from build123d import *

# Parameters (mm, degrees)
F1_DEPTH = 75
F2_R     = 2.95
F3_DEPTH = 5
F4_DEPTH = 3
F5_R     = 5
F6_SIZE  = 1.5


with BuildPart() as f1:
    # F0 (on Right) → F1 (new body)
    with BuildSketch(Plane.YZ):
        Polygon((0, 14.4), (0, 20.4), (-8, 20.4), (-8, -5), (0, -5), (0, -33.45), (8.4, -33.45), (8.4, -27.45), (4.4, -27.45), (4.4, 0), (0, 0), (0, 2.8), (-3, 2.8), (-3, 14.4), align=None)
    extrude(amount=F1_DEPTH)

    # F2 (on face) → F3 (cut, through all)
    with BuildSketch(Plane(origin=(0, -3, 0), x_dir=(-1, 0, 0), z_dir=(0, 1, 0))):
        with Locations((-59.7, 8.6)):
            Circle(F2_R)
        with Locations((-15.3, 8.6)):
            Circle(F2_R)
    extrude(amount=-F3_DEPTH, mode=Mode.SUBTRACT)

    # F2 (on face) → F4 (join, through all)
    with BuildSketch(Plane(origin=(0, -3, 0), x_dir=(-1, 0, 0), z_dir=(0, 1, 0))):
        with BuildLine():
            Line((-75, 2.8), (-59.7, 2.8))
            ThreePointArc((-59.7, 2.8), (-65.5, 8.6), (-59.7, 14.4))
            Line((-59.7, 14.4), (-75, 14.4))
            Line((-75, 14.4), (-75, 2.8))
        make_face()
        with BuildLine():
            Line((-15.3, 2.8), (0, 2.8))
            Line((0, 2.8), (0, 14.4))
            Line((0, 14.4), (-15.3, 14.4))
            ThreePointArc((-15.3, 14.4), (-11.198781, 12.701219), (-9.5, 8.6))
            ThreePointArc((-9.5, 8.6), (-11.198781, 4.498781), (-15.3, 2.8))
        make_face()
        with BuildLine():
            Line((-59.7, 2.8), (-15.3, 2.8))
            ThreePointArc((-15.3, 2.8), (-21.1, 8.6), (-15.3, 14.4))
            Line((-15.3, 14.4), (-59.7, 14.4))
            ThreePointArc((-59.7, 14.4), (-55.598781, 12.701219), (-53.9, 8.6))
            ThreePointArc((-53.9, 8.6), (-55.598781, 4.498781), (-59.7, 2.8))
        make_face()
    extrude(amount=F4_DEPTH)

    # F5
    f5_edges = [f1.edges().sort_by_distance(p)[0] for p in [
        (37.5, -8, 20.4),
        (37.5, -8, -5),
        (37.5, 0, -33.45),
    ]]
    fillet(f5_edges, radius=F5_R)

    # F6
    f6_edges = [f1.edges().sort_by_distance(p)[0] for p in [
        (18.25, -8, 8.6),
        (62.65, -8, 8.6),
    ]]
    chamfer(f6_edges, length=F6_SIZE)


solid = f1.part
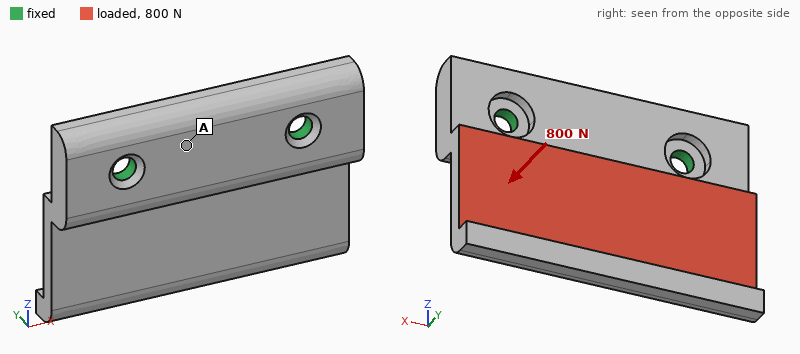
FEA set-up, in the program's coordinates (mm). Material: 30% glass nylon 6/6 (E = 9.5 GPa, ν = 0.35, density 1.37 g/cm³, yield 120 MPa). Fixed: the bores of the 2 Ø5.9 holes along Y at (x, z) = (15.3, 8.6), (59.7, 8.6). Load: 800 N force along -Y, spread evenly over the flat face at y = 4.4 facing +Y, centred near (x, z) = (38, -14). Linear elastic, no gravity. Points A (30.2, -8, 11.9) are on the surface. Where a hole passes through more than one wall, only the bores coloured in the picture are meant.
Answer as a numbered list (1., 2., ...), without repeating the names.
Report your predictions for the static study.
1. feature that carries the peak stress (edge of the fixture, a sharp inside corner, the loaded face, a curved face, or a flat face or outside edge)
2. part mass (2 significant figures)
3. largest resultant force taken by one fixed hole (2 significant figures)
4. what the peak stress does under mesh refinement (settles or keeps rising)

1. edge of the fixture
2. 36 g
3. 410 N
4. keeps rising
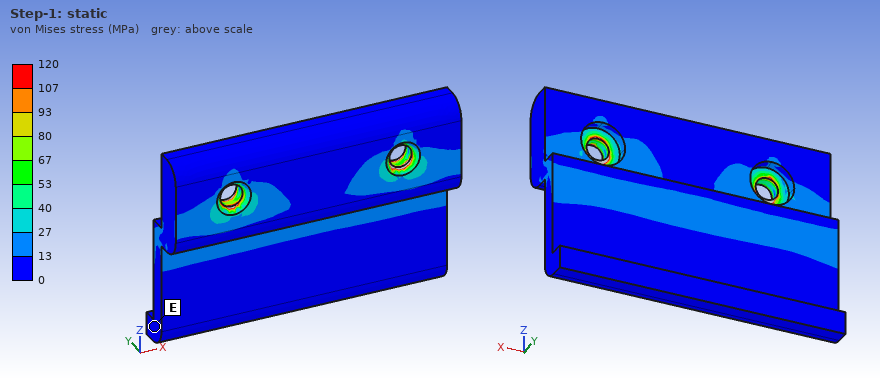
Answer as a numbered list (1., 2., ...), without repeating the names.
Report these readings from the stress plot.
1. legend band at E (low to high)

1. 0 to 13 MPa
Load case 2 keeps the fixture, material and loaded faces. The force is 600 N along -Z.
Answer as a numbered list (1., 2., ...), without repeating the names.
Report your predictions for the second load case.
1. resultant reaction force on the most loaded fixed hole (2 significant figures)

1. 300 N
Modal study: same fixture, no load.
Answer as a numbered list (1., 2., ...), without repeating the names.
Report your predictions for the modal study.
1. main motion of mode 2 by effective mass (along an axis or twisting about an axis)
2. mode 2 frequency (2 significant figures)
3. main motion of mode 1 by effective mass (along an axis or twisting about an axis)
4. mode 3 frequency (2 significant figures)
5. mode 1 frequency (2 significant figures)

1. twisting about Z
2. 1800 Hz
3. along Y
4. 4200 Hz
5. 1000 Hz
